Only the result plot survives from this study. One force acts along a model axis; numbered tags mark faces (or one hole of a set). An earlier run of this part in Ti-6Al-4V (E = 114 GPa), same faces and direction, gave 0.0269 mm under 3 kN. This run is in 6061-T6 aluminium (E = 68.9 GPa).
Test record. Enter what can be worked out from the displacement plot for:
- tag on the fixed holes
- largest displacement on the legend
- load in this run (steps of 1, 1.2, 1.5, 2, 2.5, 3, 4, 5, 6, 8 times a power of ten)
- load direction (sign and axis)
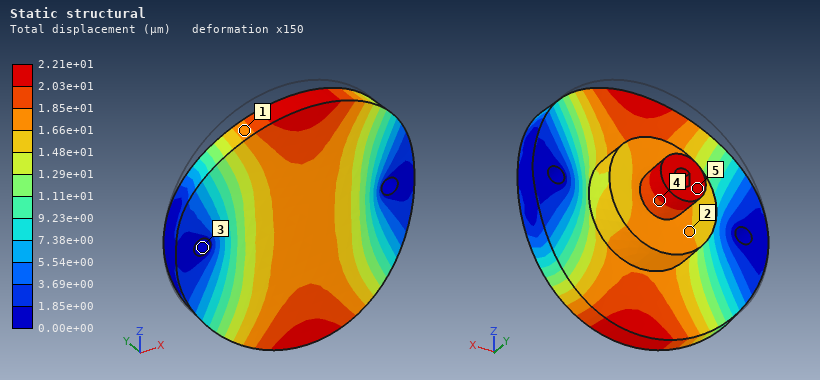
3
2.21e+01 µm
1.5 kN
-Y
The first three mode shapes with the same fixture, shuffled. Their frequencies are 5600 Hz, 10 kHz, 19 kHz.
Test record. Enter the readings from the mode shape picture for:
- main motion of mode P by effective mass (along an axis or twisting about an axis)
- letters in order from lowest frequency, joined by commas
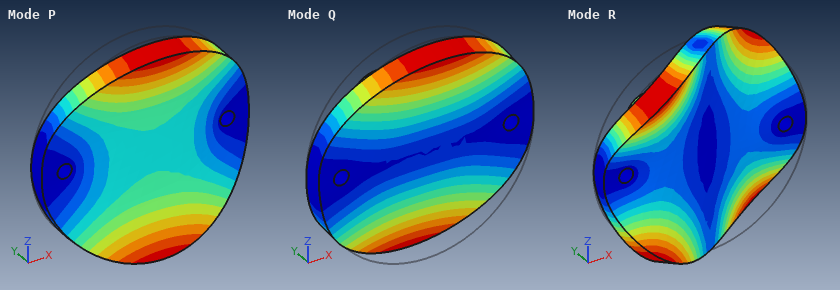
along Y
Q, P, R
